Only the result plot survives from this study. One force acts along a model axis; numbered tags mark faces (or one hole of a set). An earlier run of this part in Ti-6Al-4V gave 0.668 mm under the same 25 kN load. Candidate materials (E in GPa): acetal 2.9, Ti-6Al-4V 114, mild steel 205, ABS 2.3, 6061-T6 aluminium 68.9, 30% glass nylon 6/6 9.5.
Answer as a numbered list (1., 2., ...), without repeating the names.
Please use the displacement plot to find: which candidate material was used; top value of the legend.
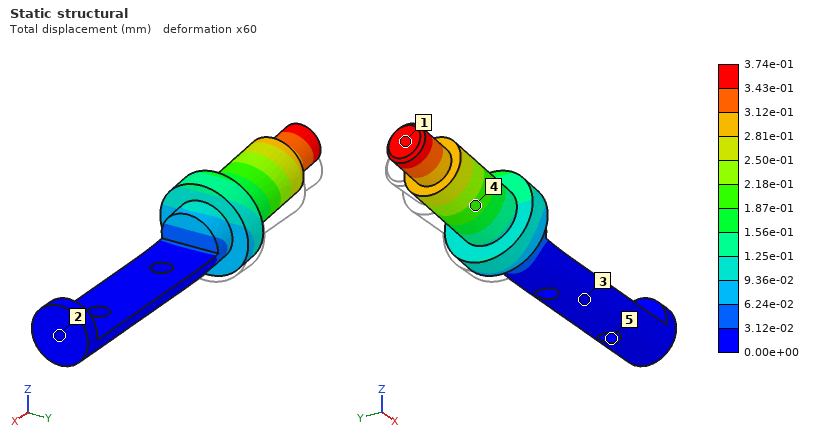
1. mild steel
2. 3.74e-01 mm
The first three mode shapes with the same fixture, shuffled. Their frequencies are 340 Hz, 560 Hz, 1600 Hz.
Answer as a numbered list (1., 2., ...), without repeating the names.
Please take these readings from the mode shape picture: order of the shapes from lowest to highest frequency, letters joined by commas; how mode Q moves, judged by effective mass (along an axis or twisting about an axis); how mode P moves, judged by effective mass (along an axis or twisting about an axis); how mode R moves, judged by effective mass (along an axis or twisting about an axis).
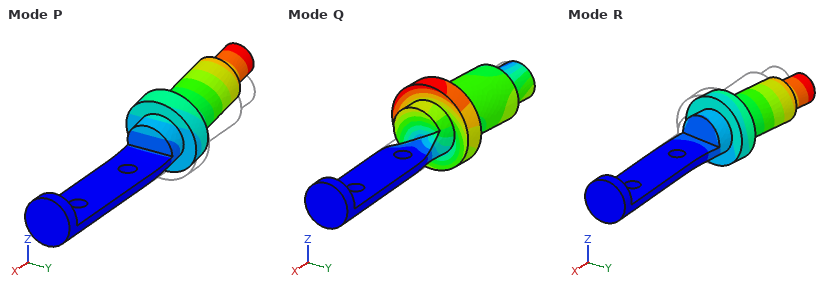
1. P, R, Q
2. twisting about X
3. along Z
4. along Y
